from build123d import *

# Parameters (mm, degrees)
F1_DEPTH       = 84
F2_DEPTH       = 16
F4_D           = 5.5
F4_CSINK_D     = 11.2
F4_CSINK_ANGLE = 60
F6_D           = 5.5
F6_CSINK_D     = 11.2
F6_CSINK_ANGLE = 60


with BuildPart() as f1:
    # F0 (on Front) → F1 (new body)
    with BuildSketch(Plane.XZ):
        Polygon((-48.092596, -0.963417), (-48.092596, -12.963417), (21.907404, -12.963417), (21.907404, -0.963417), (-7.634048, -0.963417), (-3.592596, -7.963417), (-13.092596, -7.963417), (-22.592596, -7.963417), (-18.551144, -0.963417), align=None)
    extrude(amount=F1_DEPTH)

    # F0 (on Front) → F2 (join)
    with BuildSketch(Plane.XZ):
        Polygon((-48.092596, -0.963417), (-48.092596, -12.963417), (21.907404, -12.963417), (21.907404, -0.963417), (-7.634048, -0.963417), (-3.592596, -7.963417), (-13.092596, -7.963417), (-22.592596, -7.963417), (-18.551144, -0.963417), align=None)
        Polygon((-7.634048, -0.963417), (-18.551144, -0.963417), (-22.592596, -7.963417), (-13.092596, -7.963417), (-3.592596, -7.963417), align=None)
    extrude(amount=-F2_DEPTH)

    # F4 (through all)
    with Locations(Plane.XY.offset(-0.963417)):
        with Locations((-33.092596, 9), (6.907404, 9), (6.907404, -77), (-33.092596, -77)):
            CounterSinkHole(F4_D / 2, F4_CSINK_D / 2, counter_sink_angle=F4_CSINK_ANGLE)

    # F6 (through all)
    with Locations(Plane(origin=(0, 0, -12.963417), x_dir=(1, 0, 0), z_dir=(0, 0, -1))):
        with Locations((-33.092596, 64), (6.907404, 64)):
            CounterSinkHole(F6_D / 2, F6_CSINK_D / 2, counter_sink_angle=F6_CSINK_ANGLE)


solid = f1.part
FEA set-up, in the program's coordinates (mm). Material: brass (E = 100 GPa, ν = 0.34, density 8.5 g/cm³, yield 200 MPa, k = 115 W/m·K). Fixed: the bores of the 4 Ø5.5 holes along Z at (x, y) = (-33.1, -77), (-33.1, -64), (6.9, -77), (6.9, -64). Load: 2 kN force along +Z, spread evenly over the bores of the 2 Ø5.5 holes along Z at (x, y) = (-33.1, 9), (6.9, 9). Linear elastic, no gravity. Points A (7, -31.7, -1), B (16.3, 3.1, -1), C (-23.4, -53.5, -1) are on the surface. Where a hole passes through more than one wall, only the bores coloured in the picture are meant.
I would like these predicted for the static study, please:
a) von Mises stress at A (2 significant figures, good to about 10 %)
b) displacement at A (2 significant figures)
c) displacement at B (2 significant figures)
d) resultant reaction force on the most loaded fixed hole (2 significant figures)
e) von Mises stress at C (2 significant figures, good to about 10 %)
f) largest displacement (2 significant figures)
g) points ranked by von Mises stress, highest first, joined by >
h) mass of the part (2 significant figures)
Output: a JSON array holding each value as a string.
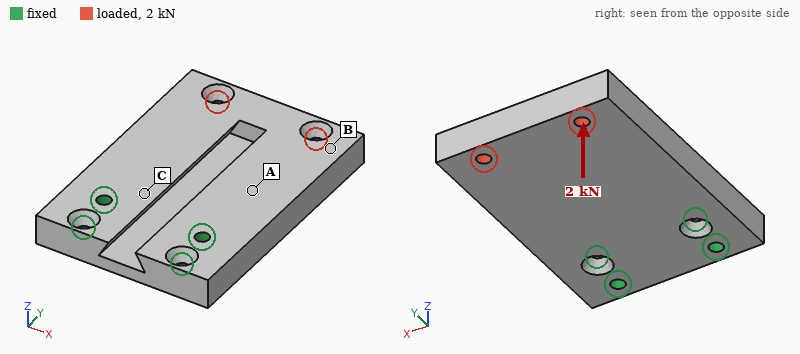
["56 MPa", "0.11 mm", "0.32 mm", "4.0 kN", "82 MPa", "0.41 mm", "C > A > B", "620 g"]
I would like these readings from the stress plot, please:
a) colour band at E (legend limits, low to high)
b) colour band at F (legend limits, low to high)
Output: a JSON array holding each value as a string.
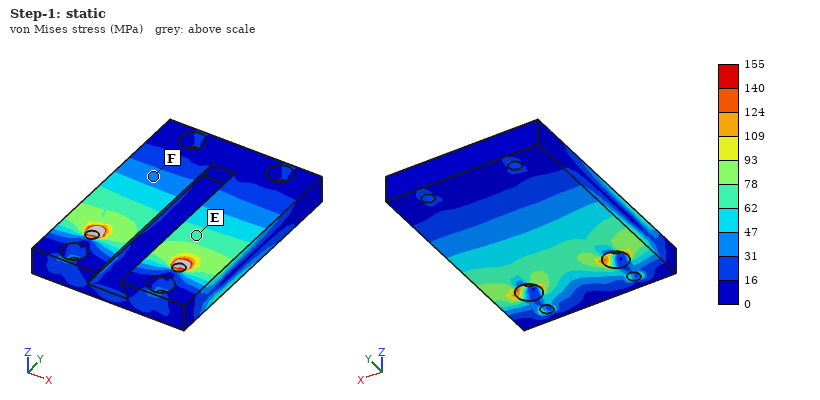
["62 to 78 MPa", "31 to 47 MPa"]
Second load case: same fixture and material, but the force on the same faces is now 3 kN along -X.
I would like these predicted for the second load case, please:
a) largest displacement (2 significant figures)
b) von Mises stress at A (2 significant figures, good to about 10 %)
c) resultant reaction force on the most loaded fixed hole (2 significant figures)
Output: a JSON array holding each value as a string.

["38 µm", "11 MPa", "3.9 kN"]
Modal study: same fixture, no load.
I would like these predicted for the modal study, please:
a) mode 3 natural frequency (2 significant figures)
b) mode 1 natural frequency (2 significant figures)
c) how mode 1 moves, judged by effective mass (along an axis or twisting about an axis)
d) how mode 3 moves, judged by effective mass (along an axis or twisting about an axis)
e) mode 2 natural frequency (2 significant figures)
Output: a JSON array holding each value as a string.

["3300 Hz", "890 Hz", "along Z", "along X", "2100 Hz"]
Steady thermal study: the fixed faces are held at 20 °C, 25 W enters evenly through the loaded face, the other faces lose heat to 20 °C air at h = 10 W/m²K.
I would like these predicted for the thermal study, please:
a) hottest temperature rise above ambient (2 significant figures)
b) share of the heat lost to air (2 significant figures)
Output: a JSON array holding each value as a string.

["25 K", "7.9 %"]
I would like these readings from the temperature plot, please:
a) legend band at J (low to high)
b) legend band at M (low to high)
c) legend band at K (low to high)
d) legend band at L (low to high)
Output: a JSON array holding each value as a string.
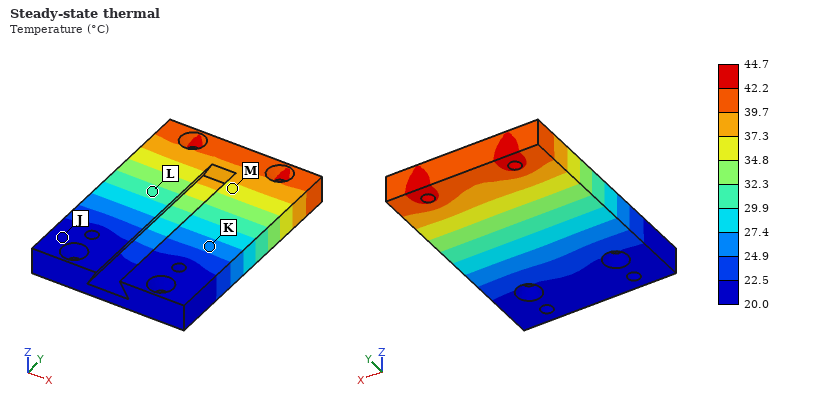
["20.0 to 22.5 °C", "34.8 to 37.3 °C", "24.9 to 27.4 °C", "29.9 to 32.3 °C"]
